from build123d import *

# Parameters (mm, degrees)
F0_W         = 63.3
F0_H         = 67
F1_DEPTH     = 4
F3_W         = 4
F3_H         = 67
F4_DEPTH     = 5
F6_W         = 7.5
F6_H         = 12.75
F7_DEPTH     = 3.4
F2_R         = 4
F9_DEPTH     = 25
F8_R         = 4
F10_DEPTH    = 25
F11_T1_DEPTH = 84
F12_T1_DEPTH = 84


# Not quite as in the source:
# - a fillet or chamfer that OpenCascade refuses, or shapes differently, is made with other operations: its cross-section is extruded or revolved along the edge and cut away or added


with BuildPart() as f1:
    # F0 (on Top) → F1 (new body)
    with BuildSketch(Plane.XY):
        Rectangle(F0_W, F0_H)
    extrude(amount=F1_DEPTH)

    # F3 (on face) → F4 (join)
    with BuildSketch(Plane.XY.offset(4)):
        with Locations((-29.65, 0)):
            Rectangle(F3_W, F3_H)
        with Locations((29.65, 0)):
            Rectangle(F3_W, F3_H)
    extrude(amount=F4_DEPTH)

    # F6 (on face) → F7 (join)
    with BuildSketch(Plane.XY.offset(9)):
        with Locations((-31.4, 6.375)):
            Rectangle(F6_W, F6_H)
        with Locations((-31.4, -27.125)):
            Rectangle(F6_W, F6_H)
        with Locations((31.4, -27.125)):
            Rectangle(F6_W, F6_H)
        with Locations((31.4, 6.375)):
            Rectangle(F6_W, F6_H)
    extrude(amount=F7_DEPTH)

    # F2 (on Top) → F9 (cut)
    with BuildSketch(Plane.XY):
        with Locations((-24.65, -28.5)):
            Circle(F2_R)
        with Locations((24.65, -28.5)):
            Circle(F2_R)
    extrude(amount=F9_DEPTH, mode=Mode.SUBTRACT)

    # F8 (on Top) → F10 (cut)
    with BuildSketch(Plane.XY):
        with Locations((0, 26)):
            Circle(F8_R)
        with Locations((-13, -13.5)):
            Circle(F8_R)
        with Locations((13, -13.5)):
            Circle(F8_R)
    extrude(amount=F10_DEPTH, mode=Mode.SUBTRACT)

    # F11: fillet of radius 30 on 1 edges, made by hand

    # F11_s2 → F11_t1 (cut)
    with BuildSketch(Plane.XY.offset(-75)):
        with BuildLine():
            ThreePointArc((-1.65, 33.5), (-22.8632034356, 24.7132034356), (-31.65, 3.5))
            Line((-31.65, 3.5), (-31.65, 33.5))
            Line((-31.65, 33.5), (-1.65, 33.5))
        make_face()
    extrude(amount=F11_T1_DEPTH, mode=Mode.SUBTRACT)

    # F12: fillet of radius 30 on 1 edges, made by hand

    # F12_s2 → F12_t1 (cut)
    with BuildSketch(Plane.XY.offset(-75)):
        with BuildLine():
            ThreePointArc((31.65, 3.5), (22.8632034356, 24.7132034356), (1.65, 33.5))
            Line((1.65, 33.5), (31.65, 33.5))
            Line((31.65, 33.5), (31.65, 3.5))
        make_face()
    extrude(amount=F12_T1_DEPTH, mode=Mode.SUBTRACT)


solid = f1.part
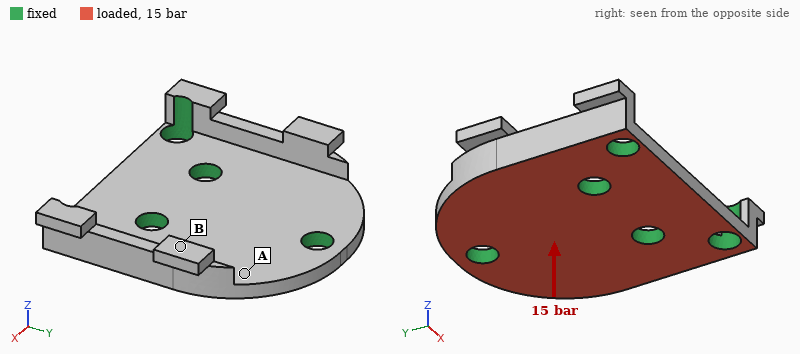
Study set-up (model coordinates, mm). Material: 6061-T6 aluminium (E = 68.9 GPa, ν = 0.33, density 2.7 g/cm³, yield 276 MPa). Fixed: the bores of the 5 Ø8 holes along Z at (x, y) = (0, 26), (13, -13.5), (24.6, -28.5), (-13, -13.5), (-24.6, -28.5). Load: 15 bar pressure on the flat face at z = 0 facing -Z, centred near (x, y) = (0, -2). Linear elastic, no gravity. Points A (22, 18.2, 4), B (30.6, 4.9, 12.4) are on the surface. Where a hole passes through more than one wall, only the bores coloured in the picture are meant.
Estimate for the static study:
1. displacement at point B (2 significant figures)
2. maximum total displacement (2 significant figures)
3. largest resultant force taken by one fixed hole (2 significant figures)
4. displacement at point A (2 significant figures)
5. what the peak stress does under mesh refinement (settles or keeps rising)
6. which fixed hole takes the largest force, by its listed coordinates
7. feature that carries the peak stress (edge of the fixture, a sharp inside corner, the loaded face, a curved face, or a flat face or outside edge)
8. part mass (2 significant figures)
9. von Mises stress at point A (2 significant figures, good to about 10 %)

0.074 mm
0.10 mm
1.6 kN
0.071 mm
keeps rising
(0, 26)
edge of the fixture
47 g
33 MPa
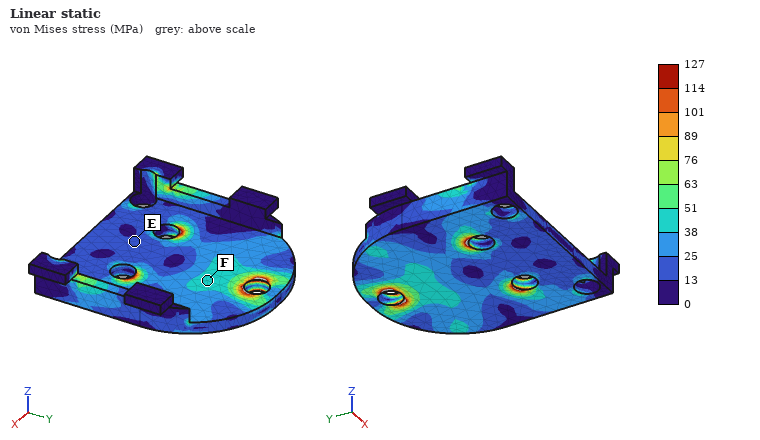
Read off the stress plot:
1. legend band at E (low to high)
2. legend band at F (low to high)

13 to 25 MPa
38 to 51 MPa
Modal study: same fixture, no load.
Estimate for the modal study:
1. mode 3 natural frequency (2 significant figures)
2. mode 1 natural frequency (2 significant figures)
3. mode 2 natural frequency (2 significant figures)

13 kHz
6200 Hz
6300 Hz
